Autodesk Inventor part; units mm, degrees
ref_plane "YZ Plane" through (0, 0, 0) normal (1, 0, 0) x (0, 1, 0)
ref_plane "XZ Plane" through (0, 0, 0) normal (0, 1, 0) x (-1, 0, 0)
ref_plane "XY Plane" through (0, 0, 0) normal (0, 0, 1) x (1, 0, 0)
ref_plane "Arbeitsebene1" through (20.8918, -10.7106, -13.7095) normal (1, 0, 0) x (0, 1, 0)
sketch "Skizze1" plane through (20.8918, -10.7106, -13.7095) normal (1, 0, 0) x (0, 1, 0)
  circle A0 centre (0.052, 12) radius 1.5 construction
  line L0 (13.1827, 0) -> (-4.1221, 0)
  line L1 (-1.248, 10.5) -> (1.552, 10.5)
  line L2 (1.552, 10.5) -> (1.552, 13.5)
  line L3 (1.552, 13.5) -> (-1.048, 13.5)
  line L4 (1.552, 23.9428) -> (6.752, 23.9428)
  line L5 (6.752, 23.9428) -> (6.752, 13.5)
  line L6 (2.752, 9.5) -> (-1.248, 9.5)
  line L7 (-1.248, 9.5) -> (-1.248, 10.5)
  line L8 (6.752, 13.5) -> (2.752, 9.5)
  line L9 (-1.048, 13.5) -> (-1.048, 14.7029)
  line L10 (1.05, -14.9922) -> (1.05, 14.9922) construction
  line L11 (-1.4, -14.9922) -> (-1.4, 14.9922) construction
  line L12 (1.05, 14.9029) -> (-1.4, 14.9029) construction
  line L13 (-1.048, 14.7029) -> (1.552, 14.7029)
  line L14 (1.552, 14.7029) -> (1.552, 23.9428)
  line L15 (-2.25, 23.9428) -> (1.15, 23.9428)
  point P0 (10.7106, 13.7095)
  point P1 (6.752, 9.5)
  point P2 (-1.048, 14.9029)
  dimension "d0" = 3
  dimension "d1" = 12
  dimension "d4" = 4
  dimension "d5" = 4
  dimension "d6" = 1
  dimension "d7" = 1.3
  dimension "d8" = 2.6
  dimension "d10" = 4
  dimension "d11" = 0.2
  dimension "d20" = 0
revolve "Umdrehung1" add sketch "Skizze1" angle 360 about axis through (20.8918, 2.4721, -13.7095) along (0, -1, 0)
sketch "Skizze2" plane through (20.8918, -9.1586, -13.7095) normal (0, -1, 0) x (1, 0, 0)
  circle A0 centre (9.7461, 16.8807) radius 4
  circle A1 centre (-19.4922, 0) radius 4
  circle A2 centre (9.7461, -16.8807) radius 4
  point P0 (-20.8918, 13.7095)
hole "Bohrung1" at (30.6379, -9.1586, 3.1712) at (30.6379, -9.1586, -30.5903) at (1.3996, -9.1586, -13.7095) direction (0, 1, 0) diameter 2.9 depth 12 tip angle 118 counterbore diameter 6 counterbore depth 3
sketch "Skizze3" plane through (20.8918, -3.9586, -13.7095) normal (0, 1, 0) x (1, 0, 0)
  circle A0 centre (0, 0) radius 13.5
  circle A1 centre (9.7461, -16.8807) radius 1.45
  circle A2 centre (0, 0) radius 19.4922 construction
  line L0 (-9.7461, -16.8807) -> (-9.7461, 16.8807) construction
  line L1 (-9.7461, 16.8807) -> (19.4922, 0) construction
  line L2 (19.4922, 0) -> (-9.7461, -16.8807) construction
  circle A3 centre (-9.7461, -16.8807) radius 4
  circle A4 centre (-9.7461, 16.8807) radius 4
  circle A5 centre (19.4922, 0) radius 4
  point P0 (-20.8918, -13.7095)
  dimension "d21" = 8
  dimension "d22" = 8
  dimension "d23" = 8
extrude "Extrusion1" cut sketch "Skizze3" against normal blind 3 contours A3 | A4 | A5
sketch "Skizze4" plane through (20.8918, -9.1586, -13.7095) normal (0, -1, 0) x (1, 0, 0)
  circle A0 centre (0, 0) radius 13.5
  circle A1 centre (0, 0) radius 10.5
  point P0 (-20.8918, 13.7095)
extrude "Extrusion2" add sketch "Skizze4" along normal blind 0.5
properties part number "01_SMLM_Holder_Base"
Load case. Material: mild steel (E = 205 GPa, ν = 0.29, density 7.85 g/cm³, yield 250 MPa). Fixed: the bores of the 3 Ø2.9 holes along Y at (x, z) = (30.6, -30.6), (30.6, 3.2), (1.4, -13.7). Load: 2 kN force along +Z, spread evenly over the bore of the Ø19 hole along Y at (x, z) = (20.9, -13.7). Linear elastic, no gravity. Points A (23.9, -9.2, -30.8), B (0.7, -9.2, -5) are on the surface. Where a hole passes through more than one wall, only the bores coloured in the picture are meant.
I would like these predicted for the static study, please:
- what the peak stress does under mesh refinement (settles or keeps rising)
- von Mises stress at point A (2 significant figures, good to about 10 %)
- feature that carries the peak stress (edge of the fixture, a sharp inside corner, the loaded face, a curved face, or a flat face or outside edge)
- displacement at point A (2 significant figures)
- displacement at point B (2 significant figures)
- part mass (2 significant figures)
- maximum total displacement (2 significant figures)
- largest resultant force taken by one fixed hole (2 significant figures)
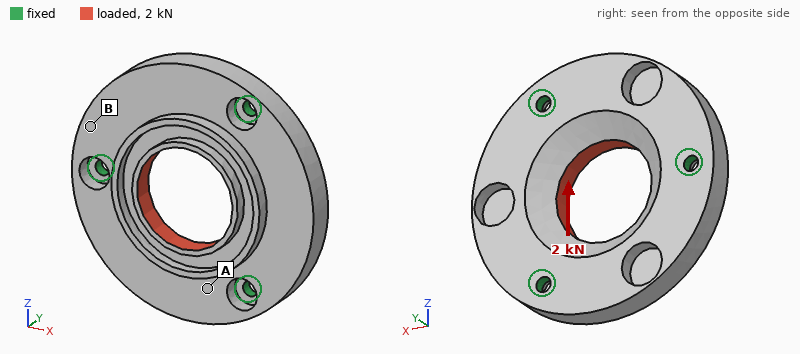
keeps rising
19 MPa
edge of the fixture
2.6 µm
4.0 µm
56 g
7.8 µm
740 N
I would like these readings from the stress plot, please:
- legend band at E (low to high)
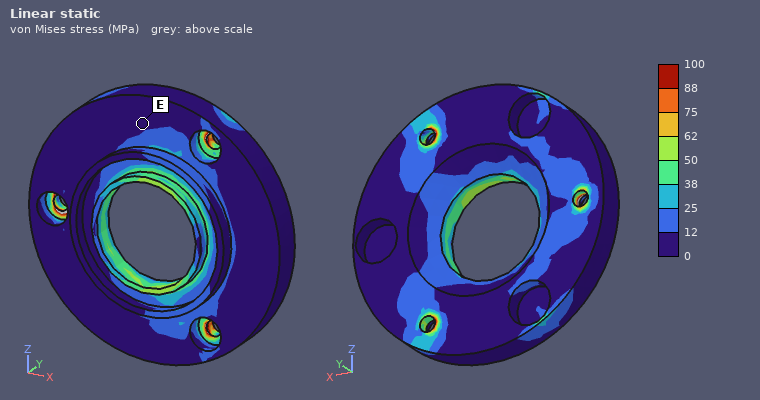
0 to 12 MPa
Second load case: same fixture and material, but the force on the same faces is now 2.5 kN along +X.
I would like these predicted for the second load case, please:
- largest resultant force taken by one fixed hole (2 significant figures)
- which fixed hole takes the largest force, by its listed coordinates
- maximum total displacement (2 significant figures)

970 N
(1.4, -13.7)
11 µm
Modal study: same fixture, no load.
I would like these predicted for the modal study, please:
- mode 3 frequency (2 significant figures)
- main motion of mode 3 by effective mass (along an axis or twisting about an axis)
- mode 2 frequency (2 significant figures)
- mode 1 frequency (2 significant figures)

14 kHz
along Y
10 kHz
10 kHz
